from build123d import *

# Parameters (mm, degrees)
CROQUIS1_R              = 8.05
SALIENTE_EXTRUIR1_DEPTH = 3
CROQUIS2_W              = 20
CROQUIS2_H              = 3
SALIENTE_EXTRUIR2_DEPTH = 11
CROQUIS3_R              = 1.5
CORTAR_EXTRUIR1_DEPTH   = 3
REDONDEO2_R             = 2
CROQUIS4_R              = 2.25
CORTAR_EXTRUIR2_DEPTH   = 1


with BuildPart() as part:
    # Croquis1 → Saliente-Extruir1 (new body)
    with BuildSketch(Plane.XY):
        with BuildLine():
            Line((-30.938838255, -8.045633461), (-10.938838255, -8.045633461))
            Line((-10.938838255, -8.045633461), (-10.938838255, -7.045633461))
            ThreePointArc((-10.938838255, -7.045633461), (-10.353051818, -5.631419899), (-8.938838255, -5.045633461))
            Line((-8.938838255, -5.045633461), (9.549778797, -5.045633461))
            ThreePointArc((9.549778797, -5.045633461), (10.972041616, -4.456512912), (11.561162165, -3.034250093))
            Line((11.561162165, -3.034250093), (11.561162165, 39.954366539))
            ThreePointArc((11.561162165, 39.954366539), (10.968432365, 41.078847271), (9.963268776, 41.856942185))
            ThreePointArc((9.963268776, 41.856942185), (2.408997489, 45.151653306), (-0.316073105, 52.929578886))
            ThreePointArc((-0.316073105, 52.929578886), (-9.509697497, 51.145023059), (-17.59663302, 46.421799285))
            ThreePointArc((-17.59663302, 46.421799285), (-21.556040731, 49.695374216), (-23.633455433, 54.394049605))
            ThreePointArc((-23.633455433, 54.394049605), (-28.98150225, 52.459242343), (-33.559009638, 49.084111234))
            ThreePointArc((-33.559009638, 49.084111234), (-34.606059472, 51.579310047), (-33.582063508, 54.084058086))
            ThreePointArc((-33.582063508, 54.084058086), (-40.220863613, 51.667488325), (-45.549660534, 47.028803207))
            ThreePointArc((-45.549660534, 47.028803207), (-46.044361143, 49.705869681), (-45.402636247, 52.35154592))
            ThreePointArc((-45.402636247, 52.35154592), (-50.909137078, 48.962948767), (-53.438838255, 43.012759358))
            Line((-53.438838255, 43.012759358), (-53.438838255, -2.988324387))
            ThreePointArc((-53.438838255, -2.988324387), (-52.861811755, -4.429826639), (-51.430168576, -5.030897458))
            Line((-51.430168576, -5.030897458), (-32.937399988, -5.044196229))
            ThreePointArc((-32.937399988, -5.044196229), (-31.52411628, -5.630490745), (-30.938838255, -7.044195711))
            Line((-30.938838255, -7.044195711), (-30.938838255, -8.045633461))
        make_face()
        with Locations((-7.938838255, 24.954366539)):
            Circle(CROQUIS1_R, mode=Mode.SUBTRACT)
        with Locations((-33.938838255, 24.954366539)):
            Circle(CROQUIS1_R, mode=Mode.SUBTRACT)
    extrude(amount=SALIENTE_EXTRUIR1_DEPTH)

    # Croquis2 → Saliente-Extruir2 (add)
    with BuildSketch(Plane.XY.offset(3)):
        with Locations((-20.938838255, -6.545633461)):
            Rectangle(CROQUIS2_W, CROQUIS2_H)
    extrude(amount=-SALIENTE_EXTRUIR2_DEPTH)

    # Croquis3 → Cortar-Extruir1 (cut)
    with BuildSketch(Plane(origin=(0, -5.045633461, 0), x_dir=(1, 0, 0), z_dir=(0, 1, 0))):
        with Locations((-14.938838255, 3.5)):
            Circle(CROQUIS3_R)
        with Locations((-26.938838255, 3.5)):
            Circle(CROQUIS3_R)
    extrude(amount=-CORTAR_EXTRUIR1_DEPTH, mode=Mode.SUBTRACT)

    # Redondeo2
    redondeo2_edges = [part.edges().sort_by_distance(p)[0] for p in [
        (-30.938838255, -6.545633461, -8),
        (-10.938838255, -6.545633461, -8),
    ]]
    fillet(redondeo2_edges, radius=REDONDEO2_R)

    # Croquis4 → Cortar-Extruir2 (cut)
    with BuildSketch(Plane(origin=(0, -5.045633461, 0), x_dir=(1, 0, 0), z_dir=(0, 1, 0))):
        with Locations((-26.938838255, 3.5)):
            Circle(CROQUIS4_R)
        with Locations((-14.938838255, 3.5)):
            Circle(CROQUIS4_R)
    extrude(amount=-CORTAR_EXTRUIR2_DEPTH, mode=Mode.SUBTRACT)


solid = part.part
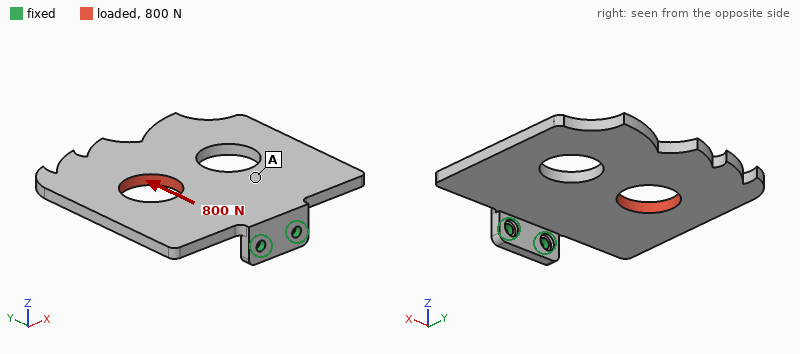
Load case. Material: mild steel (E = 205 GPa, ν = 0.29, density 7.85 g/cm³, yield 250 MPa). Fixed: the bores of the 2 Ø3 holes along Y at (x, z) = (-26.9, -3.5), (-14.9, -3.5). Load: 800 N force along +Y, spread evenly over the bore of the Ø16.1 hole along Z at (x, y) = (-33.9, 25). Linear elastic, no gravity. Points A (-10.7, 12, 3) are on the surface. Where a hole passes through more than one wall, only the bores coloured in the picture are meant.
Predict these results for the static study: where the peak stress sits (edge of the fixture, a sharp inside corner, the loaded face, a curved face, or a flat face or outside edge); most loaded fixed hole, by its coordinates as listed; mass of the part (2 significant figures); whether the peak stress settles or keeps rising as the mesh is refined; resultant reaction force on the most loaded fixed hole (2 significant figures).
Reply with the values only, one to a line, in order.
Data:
edge of the fixture
(-26.9, -3.5)
79 g
keeps rising
1.2 kN
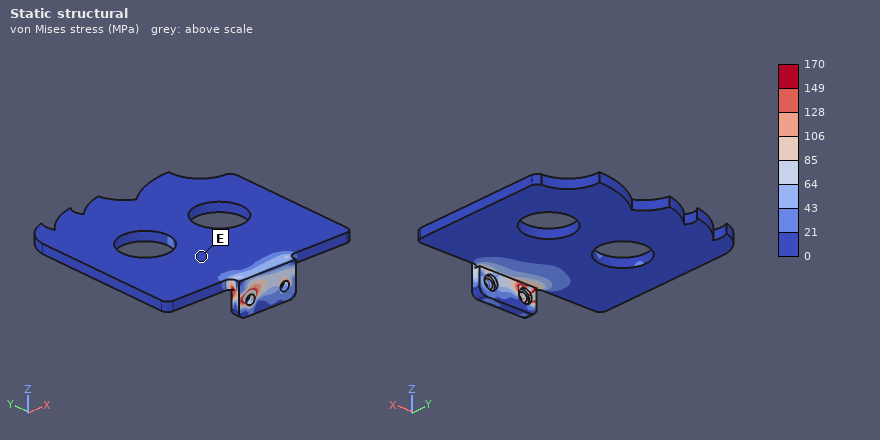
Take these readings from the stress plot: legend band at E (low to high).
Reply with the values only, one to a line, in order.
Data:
0 to 21 MPa
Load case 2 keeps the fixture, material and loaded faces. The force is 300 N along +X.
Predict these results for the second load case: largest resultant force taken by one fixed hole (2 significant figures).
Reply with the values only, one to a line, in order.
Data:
730 N
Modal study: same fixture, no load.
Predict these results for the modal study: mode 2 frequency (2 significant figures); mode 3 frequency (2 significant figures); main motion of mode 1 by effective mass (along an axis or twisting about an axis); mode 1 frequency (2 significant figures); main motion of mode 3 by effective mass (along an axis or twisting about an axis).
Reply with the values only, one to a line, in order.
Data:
1000 Hz
1600 Hz
along Z
460 Hz
along X
